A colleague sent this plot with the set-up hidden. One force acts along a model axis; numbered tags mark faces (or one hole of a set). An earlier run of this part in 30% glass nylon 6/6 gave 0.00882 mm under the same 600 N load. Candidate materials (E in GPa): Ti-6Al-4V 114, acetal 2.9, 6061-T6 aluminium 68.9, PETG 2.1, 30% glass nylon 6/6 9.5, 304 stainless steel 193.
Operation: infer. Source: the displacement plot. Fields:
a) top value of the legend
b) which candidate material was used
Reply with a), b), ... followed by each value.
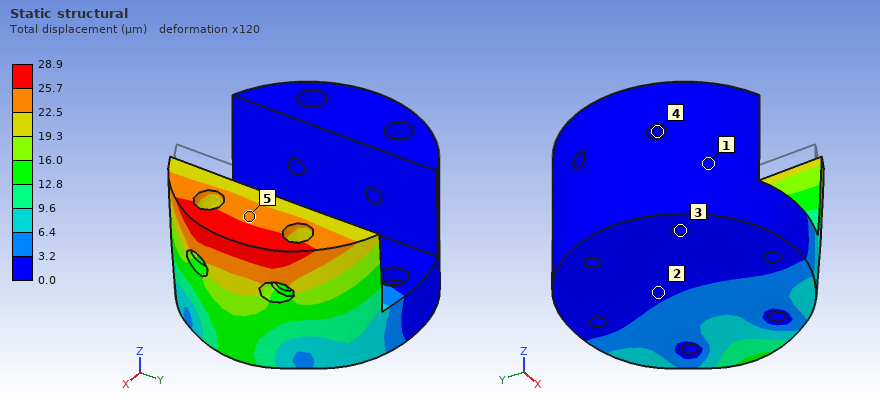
a) 28.9 µm
b) acetal
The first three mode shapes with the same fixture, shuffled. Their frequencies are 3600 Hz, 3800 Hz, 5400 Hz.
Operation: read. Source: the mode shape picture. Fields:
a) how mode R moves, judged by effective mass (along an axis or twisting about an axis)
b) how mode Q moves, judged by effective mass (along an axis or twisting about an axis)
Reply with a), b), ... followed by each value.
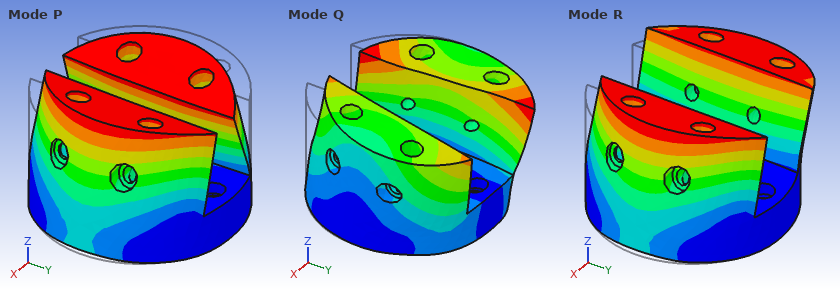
a) along X
b) along Y
